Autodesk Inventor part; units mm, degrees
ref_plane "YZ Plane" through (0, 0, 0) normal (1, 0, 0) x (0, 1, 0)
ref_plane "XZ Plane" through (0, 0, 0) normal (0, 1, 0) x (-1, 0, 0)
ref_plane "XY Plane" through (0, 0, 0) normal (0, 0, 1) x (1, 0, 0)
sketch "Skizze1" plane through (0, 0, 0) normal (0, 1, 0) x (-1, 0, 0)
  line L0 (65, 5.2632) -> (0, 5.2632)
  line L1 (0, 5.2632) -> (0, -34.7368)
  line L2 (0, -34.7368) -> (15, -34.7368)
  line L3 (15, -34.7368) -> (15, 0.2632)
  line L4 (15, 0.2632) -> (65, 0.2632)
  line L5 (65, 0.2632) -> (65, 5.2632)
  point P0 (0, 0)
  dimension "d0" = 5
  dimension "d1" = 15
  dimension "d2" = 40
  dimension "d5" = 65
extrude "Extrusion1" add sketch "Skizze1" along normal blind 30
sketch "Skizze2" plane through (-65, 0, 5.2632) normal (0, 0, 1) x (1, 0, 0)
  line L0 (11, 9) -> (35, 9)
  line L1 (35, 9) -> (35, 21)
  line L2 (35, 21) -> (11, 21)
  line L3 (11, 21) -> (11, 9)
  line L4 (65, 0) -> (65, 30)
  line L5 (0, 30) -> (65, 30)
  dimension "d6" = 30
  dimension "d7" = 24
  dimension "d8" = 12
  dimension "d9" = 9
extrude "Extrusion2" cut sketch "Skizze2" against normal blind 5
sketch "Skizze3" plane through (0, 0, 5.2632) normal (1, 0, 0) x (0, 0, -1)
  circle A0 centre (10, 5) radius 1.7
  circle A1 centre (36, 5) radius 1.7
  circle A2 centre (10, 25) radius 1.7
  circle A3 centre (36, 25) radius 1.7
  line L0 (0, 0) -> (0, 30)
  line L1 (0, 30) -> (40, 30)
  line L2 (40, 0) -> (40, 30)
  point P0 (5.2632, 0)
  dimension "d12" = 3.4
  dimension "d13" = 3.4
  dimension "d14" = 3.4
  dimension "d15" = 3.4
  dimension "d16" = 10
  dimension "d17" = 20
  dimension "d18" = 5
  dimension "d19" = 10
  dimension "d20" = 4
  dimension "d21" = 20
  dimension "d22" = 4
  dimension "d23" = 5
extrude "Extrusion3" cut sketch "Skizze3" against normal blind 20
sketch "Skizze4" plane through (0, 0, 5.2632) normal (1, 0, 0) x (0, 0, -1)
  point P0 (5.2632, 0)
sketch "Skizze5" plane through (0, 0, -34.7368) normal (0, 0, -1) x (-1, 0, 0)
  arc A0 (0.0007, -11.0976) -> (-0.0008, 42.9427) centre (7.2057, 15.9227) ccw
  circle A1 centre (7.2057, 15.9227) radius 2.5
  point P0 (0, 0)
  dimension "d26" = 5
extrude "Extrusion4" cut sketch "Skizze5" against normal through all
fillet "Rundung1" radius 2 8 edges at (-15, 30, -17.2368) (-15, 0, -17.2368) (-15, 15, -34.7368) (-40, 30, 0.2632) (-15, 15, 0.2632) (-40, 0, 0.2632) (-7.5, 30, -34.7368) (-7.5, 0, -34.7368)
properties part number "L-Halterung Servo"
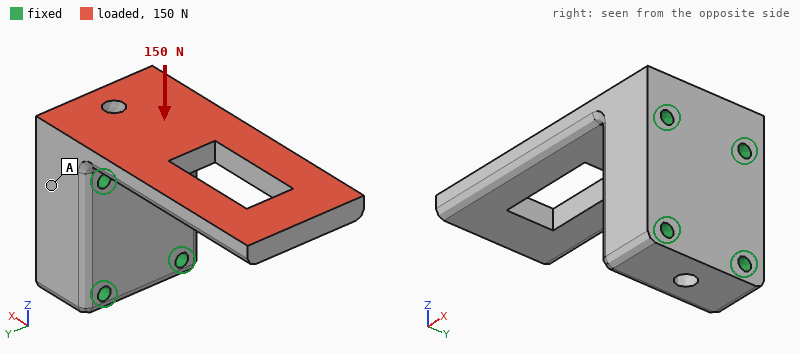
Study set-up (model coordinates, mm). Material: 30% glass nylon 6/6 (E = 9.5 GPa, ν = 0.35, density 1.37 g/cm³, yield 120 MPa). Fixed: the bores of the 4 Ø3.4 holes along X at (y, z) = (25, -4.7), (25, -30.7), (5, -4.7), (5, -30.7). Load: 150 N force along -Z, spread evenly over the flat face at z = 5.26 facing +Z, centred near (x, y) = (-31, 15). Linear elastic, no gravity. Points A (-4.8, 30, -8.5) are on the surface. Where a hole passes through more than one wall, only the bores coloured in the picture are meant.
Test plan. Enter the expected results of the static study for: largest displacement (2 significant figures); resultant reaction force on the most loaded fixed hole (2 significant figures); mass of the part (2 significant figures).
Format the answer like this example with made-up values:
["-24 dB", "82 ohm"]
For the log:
["0.84 mm", "75 N", "31 g"]
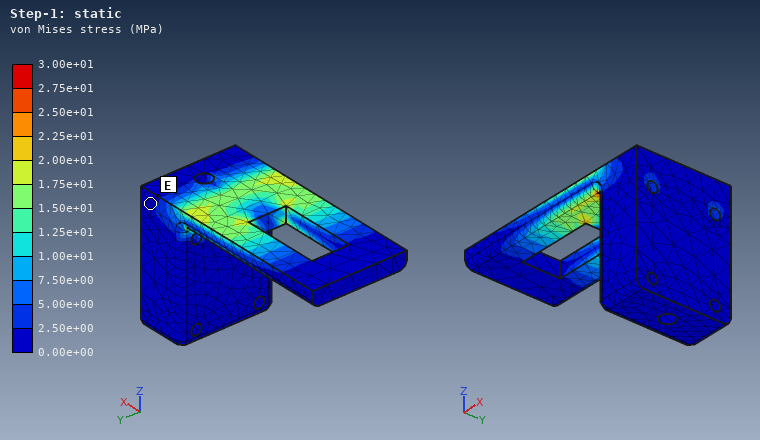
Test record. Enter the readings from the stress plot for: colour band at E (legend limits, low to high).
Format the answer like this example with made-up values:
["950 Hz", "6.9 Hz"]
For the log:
["0.00e+00 to 2.50e+00 MPa"]
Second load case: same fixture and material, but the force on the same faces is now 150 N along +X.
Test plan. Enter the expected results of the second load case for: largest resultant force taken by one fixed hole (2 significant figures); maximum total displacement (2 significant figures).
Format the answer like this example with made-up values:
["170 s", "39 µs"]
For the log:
["81 N", "0.12 mm"]
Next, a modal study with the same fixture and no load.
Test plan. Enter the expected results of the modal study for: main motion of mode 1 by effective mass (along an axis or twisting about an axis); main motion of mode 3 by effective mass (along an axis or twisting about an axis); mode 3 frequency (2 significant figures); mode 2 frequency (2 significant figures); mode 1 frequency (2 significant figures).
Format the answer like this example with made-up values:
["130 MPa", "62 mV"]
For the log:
["along Z", "along Y", "2600 Hz", "2300 Hz", "770 Hz"]
